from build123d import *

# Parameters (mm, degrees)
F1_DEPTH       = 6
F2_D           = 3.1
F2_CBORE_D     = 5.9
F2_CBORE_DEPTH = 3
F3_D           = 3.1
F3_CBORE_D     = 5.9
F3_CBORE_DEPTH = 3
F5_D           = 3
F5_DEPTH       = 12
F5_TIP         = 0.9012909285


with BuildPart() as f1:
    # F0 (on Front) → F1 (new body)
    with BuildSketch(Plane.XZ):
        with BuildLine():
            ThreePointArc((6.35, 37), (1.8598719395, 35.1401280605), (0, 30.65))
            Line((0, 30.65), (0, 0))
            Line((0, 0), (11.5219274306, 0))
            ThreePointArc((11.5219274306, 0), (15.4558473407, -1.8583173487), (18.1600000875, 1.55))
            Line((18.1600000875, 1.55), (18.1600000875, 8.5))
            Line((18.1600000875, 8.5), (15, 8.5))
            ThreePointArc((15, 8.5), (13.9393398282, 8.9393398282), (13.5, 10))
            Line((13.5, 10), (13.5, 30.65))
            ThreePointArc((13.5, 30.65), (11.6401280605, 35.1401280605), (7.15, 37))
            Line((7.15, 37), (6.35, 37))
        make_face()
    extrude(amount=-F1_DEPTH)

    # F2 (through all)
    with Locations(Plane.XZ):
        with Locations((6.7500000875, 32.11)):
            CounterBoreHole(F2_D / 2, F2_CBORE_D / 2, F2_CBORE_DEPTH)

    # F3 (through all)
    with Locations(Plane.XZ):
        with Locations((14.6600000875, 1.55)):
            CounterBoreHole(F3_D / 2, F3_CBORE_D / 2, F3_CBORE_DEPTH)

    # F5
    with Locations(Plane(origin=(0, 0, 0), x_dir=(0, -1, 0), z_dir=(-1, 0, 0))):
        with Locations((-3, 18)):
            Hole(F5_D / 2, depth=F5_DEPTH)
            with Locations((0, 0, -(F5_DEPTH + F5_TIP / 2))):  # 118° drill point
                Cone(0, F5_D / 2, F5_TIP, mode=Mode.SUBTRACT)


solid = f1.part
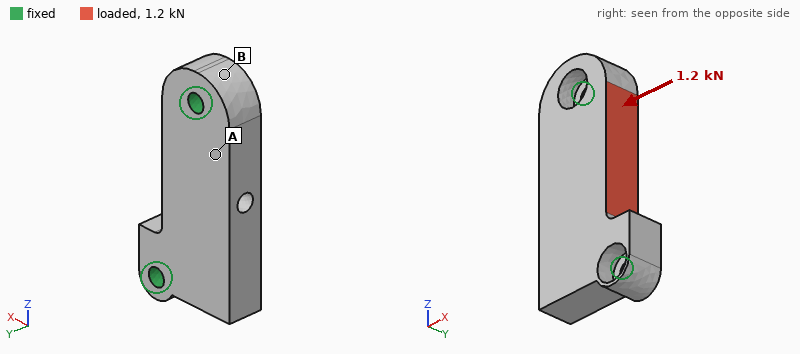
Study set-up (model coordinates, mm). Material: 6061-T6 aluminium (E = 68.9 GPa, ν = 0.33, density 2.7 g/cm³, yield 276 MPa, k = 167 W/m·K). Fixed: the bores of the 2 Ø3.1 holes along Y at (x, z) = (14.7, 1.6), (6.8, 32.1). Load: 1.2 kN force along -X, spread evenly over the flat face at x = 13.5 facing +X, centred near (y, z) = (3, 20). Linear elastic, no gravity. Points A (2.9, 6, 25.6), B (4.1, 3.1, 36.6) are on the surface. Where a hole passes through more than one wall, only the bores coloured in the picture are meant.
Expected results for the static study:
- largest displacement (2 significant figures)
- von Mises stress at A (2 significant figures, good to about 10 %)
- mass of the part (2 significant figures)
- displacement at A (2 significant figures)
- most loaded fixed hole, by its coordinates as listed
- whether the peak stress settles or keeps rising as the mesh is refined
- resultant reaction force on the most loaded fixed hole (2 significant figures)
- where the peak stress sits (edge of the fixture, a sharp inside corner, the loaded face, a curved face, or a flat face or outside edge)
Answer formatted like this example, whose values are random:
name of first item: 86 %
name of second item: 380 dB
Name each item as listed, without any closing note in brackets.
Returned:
largest displacement: 14 µm
von Mises stress at A: 17 MPa
mass of the part: 7.8 g
displacement at A: 5.8 µm
most loaded fixed hole, by its coordinates as listed: (6.8, 32.1)
whether the peak stress settles or keeps rising as the mesh is refined: keeps rising
resultant reaction force on the most loaded fixed hole: 730 N
where the peak stress sits: edge of the fixture
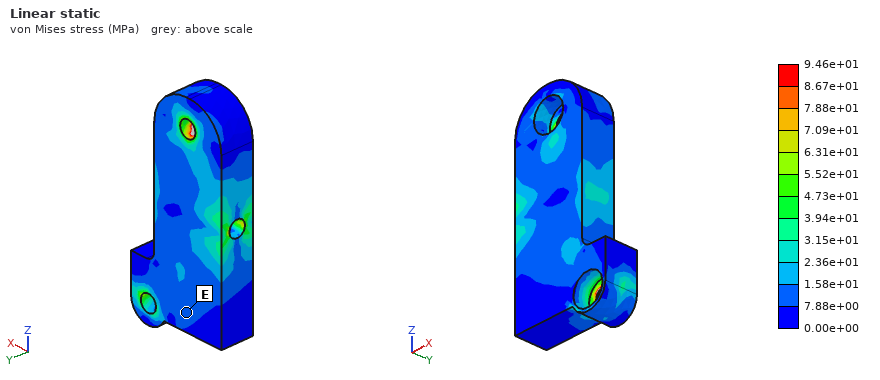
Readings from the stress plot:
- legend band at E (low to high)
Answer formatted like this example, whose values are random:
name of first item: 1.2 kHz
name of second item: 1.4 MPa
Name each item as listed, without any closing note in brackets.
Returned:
legend band at E: 7.88e+00 to 1.58e+01 MPa
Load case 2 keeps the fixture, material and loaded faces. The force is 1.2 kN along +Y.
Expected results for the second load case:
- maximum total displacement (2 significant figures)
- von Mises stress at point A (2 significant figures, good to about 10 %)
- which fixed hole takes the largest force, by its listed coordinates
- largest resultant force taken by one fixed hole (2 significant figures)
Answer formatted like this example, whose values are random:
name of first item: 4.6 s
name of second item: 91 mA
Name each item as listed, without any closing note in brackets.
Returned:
maximum total displacement: 42 µm
von Mises stress at point A: 24 MPa
which fixed hole takes the largest force, by its listed coordinates: (6.8, 32.1)
largest resultant force taken by one fixed hole: 830 N
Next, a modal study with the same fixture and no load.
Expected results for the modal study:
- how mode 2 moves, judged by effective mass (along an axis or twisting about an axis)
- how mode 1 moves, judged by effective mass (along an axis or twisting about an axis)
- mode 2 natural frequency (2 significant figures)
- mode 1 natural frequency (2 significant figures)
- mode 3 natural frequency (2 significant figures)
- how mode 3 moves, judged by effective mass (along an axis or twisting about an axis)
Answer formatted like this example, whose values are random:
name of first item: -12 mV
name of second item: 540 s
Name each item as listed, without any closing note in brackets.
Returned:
how mode 2 moves, judged by effective mass: along Y
how mode 1 moves, judged by effective mass: along Y
mode 2 natural frequency: 24 kHz
mode 1 natural frequency: 12 kHz
mode 3 natural frequency: 27 kHz
how mode 3 moves, judged by effective mass: along X
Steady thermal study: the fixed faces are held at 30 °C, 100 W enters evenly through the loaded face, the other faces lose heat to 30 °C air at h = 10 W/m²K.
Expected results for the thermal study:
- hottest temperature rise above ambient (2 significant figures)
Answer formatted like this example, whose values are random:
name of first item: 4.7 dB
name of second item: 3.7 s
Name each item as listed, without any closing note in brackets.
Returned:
hottest temperature rise above ambient: 76 K
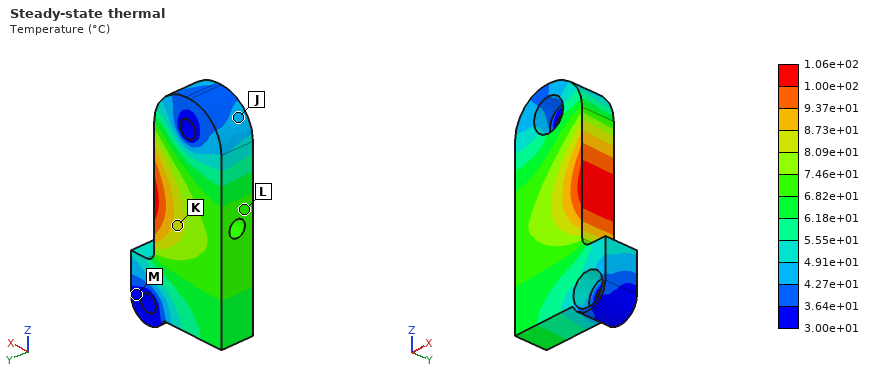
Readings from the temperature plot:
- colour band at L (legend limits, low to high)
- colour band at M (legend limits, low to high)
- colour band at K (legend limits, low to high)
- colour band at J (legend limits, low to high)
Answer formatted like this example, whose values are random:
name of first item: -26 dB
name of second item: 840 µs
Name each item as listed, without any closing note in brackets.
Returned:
colour band at L: 6.82e+01 to 7.46e+01 °C
colour band at M: 3.00e+01 to 3.64e+01 °C
colour band at K: 8.09e+01 to 8.73e+01 °C
colour band at J: 4.27e+01 to 4.91e+01 °C
